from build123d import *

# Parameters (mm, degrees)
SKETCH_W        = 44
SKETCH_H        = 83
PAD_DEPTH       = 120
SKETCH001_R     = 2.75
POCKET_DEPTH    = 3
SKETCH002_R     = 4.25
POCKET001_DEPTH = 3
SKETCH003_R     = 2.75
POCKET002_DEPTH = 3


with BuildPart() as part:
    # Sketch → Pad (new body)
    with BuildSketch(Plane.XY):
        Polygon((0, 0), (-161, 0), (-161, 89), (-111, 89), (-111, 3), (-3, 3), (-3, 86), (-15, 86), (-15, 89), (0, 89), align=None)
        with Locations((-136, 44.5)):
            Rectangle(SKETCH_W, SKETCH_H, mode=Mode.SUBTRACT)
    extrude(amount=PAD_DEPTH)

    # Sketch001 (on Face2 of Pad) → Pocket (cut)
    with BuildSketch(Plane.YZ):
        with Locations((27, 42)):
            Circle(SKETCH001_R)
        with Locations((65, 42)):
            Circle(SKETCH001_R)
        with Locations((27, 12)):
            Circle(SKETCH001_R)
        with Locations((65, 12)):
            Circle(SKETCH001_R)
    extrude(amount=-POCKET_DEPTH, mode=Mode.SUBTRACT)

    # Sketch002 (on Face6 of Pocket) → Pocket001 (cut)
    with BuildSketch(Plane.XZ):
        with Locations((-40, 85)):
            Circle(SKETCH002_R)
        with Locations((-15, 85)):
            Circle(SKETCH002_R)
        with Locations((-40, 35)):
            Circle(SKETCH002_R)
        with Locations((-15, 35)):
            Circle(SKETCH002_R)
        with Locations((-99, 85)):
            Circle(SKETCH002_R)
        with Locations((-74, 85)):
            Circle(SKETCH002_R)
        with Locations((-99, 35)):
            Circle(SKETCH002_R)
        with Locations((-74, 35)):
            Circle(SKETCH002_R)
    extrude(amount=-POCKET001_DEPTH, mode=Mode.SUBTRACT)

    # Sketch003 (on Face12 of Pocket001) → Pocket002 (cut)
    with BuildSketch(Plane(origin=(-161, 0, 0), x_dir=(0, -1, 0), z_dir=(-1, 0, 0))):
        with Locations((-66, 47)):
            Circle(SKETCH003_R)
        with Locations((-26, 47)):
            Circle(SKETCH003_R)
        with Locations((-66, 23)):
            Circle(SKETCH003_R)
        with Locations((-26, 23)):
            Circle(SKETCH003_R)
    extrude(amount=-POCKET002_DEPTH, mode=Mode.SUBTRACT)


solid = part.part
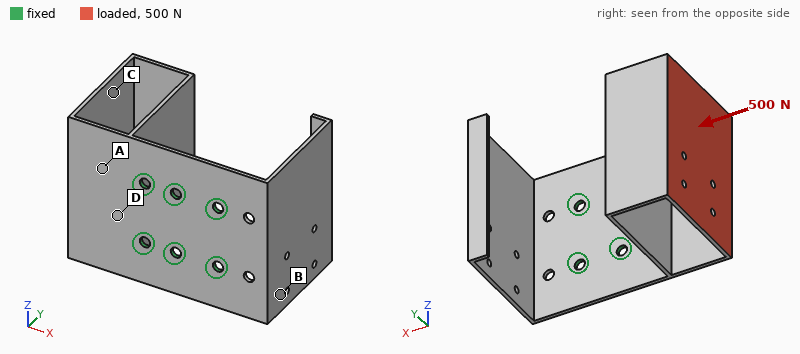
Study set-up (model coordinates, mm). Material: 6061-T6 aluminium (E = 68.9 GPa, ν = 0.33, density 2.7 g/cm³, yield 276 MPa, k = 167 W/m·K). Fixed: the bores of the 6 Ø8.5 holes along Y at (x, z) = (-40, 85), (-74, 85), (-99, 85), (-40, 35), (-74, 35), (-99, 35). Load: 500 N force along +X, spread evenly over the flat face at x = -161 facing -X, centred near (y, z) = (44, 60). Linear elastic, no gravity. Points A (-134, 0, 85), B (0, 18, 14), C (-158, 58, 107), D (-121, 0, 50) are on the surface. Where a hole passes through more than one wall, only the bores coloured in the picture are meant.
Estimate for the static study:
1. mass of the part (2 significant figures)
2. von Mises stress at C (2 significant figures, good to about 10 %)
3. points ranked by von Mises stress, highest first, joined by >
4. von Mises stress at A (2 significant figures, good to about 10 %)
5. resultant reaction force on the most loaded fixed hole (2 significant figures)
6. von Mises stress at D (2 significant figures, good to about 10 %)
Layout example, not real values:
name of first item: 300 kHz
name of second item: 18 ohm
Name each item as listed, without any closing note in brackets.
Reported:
mass of the part: 460 g
von Mises stress at C: 20 MPa
points ranked by von Mises stress, highest first, joined by >: D > A > C > B
von Mises stress at A: 33 MPa
resultant reaction force on the most loaded fixed hole: 210 N
von Mises stress at D: 43 MPa
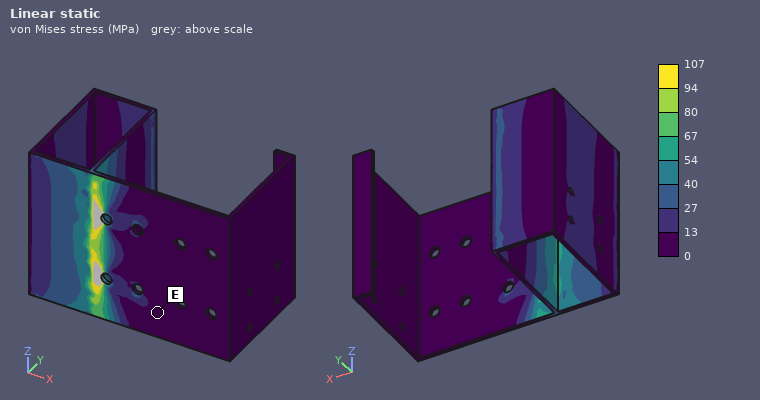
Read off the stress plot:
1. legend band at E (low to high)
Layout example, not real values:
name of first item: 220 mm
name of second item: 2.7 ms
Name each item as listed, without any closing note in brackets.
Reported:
legend band at E: 0 to 13 MPa
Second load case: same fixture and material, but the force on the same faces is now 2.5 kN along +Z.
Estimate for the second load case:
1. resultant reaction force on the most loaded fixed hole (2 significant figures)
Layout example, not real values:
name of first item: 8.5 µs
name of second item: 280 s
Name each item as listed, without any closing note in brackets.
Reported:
resultant reaction force on the most loaded fixed hole: 2.9 kN
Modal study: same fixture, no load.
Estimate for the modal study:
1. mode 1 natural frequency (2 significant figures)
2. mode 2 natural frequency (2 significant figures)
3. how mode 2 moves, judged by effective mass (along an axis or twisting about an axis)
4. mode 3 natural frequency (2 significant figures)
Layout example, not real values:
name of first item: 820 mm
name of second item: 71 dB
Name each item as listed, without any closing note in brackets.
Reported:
mode 1 natural frequency: 150 Hz
mode 2 natural frequency: 160 Hz
how mode 2 moves, judged by effective mass: along X
mode 3 natural frequency: 330 Hz
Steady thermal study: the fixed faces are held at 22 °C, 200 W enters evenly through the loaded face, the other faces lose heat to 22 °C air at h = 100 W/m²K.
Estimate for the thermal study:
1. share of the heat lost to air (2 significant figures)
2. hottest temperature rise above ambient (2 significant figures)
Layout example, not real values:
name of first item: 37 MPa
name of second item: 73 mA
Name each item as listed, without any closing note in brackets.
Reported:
share of the heat lost to air: 85 %
hottest temperature rise above ambient: 71 K
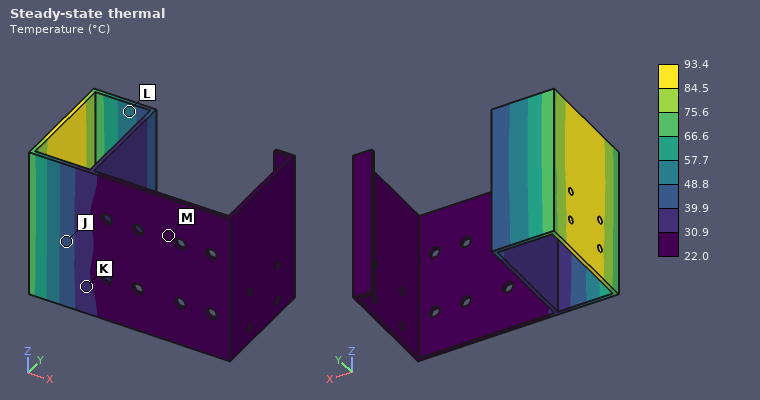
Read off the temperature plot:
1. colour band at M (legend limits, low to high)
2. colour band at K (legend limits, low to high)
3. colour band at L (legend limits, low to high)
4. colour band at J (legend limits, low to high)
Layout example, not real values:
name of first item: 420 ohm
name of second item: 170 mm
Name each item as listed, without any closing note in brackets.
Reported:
colour band at M: 22.0 to 30.9 °C
colour band at K: 30.9 to 39.9 °C
colour band at L: 48.8 to 57.7 °C
colour band at J: 39.9 to 48.8 °C
